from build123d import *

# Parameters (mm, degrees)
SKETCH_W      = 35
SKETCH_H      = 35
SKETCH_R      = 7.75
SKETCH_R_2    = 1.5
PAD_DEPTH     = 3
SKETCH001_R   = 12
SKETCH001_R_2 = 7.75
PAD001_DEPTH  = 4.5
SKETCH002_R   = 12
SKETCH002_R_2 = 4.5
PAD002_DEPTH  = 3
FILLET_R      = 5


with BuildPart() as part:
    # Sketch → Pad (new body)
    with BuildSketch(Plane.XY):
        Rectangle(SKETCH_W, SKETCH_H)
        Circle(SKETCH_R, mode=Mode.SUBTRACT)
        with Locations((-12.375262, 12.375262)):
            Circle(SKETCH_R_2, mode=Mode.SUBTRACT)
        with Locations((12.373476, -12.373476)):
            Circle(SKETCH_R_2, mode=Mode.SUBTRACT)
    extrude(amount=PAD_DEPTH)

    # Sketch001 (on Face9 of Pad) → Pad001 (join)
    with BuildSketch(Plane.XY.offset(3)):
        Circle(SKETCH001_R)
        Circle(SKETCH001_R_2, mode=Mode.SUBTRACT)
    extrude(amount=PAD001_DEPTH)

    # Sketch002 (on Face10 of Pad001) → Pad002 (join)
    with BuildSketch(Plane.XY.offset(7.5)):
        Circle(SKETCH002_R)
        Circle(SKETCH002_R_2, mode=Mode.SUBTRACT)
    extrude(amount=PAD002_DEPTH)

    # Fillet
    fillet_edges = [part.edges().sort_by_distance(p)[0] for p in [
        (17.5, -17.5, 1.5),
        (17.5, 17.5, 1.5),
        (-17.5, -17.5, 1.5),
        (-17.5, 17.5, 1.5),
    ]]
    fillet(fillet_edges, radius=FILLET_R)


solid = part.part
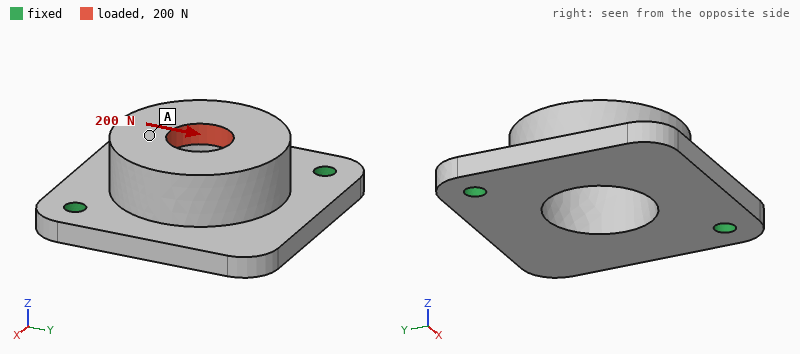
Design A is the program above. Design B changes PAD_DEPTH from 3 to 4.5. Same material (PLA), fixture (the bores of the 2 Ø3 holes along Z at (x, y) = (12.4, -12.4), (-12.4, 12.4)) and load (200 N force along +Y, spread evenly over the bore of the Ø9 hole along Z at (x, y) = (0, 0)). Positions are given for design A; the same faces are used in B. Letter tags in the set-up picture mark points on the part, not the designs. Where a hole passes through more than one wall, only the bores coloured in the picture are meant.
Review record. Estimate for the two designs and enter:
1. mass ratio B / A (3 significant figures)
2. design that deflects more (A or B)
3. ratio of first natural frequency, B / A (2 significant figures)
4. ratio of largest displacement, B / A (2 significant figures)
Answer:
1.21
A
1.4
0.36
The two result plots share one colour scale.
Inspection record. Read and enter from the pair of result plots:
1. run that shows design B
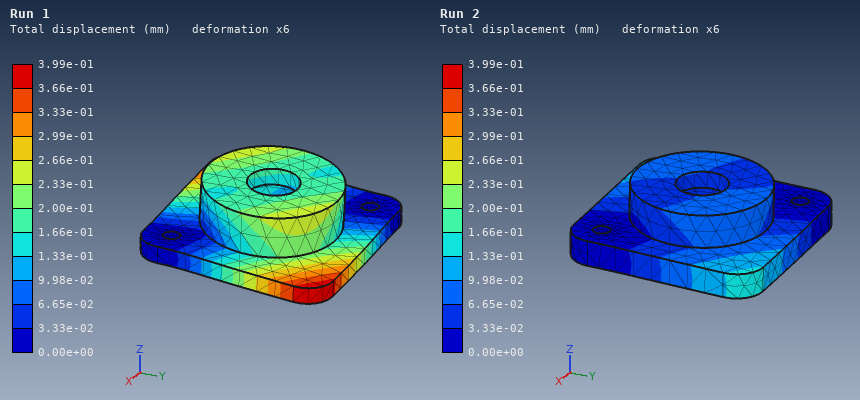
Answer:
Run 2
